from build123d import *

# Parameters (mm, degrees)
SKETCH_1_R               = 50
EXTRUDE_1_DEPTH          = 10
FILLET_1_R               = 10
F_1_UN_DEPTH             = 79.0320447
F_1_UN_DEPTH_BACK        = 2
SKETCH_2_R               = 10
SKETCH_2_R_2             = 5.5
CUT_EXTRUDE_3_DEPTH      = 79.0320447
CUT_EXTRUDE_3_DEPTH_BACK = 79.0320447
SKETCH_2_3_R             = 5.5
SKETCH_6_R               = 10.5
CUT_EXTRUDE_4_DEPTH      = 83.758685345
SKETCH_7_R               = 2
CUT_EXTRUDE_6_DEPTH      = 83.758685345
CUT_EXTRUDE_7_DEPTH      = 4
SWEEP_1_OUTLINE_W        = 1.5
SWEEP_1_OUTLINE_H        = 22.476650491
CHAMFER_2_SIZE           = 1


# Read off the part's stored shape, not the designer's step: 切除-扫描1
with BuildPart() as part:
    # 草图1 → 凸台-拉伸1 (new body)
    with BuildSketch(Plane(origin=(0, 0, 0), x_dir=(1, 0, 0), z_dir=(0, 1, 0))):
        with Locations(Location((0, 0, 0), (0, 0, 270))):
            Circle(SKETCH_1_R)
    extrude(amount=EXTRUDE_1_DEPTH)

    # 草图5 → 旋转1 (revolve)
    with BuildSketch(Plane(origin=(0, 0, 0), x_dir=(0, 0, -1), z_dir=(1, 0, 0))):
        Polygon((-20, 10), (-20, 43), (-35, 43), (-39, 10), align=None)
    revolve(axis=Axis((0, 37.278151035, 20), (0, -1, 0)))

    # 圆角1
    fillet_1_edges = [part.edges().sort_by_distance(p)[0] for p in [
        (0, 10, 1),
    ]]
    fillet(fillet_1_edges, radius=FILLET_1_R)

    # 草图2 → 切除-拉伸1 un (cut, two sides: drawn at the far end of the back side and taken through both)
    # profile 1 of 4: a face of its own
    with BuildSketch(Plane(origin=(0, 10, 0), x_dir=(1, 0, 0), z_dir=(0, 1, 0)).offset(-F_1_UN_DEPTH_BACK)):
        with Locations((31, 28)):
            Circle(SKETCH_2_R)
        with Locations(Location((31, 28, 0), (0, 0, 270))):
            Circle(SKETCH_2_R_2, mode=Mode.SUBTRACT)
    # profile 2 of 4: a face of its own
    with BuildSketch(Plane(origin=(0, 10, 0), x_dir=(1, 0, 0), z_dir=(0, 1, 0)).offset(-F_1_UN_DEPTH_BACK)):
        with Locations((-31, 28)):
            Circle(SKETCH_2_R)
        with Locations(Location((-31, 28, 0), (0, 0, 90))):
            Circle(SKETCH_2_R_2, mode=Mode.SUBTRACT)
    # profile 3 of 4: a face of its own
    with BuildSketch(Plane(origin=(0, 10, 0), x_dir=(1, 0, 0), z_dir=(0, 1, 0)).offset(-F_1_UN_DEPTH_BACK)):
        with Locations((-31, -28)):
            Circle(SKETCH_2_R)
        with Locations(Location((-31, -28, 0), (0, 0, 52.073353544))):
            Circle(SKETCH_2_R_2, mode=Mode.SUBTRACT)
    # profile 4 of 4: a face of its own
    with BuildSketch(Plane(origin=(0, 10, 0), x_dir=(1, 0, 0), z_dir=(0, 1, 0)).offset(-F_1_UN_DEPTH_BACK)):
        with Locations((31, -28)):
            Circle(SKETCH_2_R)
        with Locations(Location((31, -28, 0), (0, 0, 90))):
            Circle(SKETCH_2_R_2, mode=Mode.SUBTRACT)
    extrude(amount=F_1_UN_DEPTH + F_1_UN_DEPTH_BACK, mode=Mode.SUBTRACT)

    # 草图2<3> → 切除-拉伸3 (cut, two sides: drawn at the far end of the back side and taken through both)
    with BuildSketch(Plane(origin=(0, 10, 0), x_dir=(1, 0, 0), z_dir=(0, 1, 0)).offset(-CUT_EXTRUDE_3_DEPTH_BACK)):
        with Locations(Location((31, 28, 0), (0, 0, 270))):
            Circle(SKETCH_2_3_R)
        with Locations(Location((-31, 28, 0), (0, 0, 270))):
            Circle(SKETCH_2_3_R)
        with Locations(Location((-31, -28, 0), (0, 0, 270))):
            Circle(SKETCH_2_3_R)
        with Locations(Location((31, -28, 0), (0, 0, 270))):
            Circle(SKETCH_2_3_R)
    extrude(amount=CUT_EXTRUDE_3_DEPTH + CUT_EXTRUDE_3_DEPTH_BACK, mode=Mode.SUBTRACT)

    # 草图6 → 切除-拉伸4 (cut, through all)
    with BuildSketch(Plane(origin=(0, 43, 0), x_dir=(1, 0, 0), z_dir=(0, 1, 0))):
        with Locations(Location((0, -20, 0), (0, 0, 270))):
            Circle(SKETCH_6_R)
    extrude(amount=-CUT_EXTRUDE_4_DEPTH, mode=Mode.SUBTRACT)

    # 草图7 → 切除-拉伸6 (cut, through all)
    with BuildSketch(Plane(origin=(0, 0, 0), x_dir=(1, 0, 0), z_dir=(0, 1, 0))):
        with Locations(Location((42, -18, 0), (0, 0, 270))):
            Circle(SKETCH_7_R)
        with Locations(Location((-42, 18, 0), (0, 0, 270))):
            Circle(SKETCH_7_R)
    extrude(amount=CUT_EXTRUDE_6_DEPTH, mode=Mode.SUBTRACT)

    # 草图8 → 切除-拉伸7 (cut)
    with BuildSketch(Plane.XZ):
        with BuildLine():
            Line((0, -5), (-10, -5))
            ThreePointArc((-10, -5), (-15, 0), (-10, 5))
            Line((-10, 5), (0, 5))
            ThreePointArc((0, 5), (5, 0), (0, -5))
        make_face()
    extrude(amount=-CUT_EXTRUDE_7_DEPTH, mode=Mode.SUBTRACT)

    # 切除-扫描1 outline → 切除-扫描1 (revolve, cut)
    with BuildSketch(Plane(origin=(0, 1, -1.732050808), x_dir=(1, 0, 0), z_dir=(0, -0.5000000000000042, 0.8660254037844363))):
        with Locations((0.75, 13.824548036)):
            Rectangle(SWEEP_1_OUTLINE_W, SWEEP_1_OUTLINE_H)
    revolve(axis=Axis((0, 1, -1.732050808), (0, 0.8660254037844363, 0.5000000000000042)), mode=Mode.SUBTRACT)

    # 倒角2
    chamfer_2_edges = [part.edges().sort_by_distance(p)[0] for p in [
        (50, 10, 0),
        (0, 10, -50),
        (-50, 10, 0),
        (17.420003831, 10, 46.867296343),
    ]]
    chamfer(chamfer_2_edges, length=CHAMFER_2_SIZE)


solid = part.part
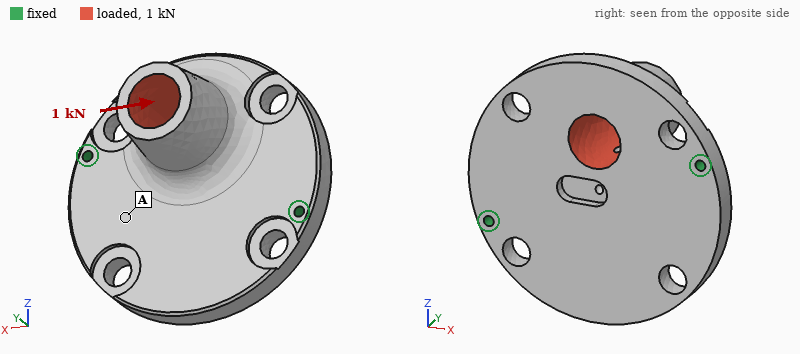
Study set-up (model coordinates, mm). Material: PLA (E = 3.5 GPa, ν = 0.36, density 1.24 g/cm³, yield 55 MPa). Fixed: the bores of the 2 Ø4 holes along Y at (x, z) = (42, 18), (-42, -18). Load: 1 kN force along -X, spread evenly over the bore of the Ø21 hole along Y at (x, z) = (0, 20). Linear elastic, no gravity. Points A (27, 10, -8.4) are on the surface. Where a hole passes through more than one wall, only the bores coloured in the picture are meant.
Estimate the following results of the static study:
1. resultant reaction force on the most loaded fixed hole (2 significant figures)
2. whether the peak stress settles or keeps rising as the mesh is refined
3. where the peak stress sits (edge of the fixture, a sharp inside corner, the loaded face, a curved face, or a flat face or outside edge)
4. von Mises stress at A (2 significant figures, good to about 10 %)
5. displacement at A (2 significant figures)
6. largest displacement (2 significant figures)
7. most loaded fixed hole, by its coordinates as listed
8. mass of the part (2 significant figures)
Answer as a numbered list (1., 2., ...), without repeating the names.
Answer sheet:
1. 630 N
2. keeps rising
3. edge of the fixture
4. 2.2 MPa
5. 0.13 mm
6. 0.53 mm
7. (42, 18)
8. 110 g
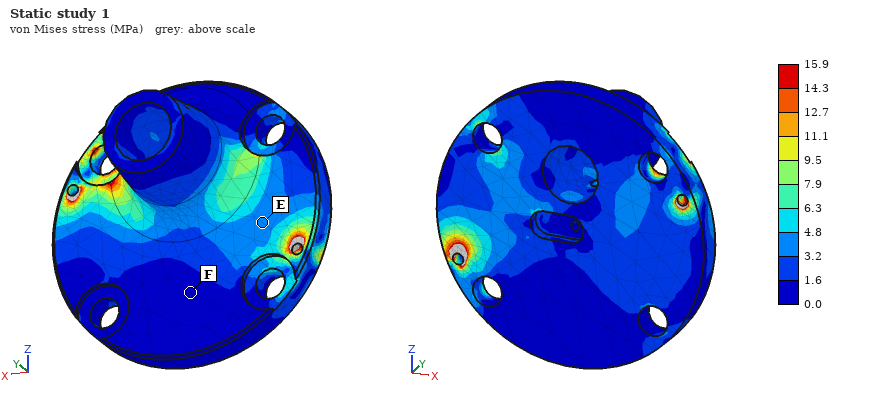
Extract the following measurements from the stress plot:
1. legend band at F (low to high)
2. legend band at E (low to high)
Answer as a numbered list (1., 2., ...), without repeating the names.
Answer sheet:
1. 0.0 to 1.6 MPa
2. 3.2 to 4.8 MPa
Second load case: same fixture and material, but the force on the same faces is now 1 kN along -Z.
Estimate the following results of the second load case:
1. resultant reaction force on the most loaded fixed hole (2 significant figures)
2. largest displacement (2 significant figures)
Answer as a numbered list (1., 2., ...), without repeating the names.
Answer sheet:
1. 520 N
2. 1.1 mm
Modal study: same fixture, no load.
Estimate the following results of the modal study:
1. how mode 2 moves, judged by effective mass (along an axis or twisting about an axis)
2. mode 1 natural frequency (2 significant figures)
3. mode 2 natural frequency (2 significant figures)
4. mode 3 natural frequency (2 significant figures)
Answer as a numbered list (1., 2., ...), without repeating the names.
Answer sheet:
1. along Y
2. 530 Hz
3. 940 Hz
4. 1900 Hz
